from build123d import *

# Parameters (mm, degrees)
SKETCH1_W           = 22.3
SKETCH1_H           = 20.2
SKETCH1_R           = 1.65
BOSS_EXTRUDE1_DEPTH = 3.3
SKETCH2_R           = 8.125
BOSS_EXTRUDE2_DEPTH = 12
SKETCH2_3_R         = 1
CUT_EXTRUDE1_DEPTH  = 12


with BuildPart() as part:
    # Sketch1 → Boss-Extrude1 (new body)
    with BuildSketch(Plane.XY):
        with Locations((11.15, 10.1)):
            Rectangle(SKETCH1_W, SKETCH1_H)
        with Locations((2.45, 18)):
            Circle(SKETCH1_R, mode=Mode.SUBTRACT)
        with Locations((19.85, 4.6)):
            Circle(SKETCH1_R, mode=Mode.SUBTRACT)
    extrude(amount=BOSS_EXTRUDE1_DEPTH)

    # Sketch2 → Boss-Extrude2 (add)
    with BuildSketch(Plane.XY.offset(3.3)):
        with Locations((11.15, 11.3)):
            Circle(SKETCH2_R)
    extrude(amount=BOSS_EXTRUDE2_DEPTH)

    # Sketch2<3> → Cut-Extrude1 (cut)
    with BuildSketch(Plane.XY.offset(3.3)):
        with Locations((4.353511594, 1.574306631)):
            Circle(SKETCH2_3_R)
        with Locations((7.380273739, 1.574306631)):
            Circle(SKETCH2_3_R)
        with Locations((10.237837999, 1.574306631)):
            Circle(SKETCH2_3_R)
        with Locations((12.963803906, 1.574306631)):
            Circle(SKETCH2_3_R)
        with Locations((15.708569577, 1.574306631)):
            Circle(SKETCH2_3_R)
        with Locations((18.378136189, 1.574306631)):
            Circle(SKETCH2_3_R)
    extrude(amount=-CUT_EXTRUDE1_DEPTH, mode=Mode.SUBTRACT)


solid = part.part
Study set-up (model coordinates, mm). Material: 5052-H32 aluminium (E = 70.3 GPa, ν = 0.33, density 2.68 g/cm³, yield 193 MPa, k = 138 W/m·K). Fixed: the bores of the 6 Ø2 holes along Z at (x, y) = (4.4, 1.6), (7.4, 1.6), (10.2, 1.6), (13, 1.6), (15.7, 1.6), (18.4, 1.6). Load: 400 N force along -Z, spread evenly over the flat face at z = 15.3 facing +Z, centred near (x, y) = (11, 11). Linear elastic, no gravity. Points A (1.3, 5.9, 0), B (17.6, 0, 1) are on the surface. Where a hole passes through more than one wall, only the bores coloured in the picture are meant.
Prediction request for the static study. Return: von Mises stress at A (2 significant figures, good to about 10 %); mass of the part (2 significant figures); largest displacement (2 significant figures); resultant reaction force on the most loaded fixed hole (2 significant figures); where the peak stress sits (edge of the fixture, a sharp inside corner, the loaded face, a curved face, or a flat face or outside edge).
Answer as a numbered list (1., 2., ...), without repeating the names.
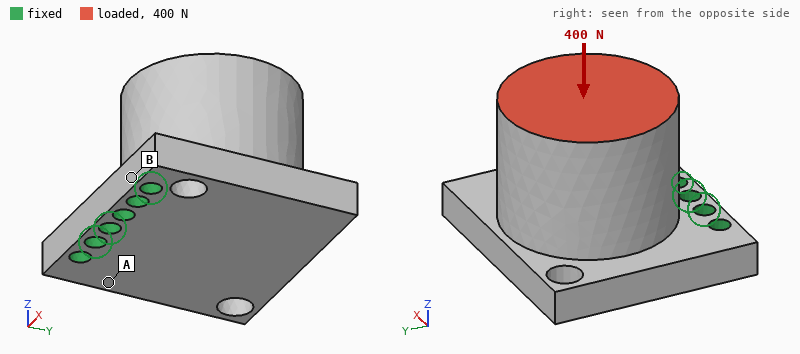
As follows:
1. 31 MPa
2. 10 g
3. 55 µm
4. 100 N
5. edge of the fixture
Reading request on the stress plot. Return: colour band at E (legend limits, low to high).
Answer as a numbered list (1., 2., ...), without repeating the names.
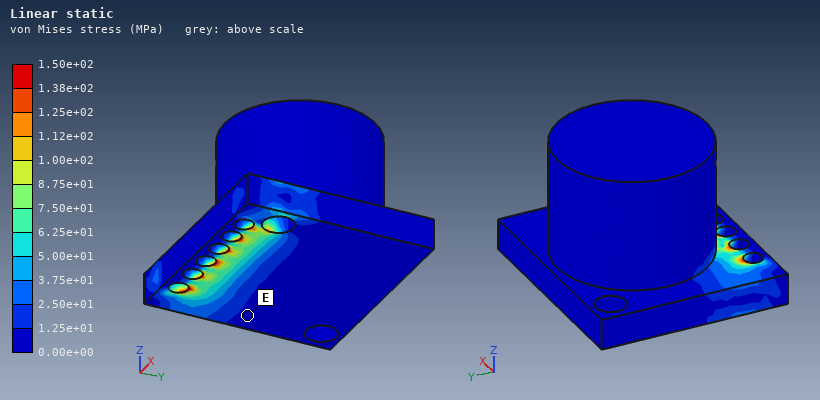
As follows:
1. 0.00e+00 to 1.25e+01 MPa
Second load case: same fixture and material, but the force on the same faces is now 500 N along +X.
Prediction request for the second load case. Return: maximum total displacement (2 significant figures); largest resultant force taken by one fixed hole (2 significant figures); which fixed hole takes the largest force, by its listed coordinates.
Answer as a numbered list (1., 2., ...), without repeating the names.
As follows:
1. 27 µm
2. 410 N
3. (4.4, 1.6)
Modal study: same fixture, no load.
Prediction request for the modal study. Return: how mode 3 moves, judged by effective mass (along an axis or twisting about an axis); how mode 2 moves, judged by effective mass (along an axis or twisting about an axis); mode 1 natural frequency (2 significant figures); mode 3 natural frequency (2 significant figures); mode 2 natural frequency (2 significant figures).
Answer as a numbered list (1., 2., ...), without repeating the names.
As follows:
1. along X
2. along X
3. 4900 Hz
4. 20 kHz
5. 12 kHz
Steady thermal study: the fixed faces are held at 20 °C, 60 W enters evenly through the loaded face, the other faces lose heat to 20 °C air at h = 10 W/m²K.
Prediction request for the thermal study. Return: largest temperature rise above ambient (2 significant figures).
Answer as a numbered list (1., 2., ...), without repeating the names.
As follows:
1. 62 K
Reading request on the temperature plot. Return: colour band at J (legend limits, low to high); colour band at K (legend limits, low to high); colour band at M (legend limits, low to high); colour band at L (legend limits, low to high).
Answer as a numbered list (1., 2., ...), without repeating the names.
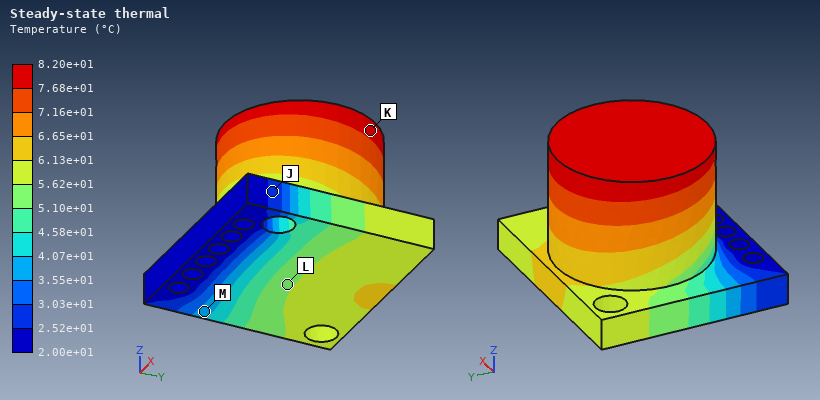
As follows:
1. 2.52e+01 to 3.03e+01 °C
2. 7.68e+01 to 8.20e+01 °C
3. 3.55e+01 to 4.07e+01 °C
4. 5.10e+01 to 5.62e+01 °C
